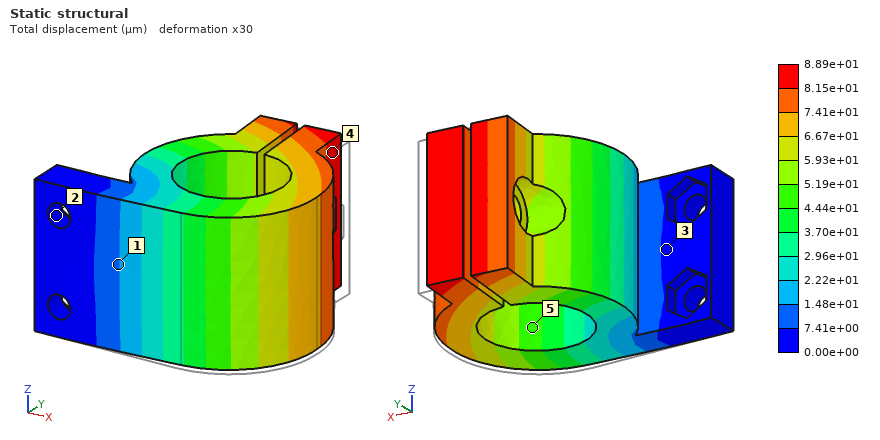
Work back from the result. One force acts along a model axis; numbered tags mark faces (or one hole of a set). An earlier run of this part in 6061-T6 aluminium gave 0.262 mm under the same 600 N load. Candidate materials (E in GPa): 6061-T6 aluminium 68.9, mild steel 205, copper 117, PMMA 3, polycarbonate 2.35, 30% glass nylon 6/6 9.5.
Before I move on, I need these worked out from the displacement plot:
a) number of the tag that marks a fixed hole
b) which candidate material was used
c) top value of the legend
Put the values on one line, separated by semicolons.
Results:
2; mild steel; 8.89e+01 µm
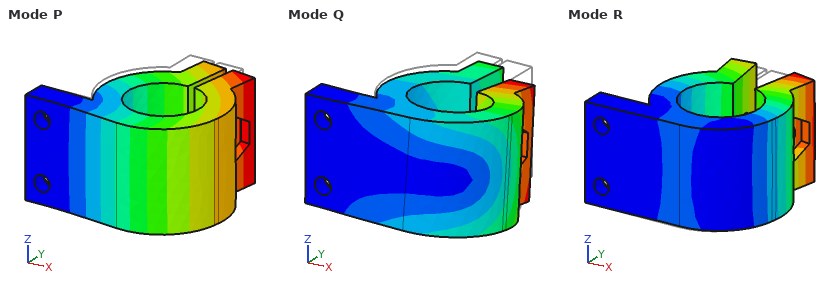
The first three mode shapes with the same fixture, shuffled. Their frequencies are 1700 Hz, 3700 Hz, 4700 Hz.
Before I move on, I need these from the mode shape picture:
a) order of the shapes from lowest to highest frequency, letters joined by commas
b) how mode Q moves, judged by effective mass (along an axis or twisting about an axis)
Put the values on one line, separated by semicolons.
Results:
P, Q, R; along Z
